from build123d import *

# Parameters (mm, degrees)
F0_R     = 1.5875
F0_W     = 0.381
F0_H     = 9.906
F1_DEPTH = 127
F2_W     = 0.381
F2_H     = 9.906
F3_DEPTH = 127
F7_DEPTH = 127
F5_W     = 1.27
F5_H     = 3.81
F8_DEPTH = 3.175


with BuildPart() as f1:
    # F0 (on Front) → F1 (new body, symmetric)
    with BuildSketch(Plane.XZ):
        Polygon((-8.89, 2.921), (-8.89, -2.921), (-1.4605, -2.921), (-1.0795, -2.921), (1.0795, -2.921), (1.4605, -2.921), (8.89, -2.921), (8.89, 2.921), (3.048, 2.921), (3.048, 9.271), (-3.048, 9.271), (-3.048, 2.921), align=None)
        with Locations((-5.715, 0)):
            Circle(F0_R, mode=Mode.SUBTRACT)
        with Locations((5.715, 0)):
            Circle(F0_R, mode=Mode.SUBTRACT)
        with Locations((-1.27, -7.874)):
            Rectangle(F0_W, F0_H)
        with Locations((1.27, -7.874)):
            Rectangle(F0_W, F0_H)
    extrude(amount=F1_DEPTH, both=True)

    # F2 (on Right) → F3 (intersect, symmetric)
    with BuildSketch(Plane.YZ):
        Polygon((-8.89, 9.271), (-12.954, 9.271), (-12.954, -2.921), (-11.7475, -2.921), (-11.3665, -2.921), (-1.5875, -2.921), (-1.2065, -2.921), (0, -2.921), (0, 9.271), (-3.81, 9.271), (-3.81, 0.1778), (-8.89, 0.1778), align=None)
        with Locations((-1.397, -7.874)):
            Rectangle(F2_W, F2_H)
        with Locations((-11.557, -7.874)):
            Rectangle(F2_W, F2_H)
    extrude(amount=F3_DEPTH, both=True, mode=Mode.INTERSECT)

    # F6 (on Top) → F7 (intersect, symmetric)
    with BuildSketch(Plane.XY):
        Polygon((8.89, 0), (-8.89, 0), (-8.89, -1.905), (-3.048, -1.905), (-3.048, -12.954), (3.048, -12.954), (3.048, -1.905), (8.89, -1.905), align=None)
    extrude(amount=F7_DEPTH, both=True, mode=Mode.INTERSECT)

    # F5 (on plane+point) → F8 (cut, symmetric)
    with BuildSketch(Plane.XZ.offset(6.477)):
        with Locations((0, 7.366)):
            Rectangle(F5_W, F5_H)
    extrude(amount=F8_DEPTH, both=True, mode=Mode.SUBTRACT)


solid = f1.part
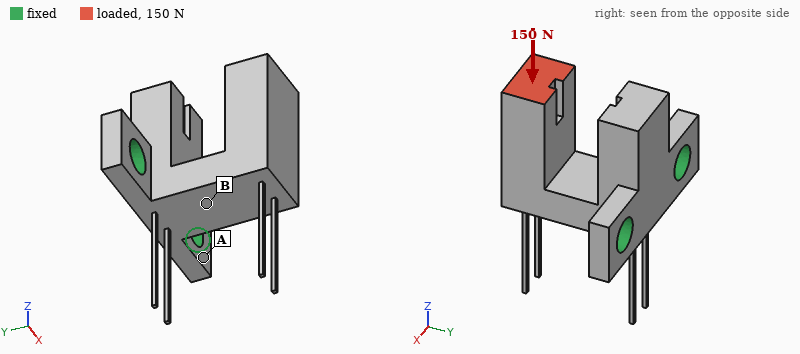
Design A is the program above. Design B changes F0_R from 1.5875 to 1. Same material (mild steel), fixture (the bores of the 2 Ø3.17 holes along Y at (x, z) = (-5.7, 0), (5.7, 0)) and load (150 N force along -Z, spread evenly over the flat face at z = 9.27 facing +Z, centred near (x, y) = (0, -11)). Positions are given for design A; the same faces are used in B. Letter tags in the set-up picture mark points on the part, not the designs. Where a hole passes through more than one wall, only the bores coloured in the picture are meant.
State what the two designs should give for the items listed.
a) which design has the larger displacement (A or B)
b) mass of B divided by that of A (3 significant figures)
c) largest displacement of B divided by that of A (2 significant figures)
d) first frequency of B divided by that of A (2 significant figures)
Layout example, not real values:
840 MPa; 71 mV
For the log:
B; 1.02; 1.2; 1.0
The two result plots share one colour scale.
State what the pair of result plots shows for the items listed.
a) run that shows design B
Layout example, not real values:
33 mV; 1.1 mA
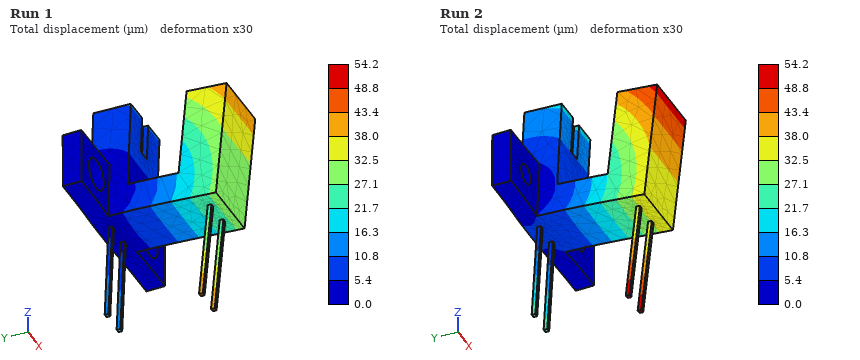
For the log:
Run 2
